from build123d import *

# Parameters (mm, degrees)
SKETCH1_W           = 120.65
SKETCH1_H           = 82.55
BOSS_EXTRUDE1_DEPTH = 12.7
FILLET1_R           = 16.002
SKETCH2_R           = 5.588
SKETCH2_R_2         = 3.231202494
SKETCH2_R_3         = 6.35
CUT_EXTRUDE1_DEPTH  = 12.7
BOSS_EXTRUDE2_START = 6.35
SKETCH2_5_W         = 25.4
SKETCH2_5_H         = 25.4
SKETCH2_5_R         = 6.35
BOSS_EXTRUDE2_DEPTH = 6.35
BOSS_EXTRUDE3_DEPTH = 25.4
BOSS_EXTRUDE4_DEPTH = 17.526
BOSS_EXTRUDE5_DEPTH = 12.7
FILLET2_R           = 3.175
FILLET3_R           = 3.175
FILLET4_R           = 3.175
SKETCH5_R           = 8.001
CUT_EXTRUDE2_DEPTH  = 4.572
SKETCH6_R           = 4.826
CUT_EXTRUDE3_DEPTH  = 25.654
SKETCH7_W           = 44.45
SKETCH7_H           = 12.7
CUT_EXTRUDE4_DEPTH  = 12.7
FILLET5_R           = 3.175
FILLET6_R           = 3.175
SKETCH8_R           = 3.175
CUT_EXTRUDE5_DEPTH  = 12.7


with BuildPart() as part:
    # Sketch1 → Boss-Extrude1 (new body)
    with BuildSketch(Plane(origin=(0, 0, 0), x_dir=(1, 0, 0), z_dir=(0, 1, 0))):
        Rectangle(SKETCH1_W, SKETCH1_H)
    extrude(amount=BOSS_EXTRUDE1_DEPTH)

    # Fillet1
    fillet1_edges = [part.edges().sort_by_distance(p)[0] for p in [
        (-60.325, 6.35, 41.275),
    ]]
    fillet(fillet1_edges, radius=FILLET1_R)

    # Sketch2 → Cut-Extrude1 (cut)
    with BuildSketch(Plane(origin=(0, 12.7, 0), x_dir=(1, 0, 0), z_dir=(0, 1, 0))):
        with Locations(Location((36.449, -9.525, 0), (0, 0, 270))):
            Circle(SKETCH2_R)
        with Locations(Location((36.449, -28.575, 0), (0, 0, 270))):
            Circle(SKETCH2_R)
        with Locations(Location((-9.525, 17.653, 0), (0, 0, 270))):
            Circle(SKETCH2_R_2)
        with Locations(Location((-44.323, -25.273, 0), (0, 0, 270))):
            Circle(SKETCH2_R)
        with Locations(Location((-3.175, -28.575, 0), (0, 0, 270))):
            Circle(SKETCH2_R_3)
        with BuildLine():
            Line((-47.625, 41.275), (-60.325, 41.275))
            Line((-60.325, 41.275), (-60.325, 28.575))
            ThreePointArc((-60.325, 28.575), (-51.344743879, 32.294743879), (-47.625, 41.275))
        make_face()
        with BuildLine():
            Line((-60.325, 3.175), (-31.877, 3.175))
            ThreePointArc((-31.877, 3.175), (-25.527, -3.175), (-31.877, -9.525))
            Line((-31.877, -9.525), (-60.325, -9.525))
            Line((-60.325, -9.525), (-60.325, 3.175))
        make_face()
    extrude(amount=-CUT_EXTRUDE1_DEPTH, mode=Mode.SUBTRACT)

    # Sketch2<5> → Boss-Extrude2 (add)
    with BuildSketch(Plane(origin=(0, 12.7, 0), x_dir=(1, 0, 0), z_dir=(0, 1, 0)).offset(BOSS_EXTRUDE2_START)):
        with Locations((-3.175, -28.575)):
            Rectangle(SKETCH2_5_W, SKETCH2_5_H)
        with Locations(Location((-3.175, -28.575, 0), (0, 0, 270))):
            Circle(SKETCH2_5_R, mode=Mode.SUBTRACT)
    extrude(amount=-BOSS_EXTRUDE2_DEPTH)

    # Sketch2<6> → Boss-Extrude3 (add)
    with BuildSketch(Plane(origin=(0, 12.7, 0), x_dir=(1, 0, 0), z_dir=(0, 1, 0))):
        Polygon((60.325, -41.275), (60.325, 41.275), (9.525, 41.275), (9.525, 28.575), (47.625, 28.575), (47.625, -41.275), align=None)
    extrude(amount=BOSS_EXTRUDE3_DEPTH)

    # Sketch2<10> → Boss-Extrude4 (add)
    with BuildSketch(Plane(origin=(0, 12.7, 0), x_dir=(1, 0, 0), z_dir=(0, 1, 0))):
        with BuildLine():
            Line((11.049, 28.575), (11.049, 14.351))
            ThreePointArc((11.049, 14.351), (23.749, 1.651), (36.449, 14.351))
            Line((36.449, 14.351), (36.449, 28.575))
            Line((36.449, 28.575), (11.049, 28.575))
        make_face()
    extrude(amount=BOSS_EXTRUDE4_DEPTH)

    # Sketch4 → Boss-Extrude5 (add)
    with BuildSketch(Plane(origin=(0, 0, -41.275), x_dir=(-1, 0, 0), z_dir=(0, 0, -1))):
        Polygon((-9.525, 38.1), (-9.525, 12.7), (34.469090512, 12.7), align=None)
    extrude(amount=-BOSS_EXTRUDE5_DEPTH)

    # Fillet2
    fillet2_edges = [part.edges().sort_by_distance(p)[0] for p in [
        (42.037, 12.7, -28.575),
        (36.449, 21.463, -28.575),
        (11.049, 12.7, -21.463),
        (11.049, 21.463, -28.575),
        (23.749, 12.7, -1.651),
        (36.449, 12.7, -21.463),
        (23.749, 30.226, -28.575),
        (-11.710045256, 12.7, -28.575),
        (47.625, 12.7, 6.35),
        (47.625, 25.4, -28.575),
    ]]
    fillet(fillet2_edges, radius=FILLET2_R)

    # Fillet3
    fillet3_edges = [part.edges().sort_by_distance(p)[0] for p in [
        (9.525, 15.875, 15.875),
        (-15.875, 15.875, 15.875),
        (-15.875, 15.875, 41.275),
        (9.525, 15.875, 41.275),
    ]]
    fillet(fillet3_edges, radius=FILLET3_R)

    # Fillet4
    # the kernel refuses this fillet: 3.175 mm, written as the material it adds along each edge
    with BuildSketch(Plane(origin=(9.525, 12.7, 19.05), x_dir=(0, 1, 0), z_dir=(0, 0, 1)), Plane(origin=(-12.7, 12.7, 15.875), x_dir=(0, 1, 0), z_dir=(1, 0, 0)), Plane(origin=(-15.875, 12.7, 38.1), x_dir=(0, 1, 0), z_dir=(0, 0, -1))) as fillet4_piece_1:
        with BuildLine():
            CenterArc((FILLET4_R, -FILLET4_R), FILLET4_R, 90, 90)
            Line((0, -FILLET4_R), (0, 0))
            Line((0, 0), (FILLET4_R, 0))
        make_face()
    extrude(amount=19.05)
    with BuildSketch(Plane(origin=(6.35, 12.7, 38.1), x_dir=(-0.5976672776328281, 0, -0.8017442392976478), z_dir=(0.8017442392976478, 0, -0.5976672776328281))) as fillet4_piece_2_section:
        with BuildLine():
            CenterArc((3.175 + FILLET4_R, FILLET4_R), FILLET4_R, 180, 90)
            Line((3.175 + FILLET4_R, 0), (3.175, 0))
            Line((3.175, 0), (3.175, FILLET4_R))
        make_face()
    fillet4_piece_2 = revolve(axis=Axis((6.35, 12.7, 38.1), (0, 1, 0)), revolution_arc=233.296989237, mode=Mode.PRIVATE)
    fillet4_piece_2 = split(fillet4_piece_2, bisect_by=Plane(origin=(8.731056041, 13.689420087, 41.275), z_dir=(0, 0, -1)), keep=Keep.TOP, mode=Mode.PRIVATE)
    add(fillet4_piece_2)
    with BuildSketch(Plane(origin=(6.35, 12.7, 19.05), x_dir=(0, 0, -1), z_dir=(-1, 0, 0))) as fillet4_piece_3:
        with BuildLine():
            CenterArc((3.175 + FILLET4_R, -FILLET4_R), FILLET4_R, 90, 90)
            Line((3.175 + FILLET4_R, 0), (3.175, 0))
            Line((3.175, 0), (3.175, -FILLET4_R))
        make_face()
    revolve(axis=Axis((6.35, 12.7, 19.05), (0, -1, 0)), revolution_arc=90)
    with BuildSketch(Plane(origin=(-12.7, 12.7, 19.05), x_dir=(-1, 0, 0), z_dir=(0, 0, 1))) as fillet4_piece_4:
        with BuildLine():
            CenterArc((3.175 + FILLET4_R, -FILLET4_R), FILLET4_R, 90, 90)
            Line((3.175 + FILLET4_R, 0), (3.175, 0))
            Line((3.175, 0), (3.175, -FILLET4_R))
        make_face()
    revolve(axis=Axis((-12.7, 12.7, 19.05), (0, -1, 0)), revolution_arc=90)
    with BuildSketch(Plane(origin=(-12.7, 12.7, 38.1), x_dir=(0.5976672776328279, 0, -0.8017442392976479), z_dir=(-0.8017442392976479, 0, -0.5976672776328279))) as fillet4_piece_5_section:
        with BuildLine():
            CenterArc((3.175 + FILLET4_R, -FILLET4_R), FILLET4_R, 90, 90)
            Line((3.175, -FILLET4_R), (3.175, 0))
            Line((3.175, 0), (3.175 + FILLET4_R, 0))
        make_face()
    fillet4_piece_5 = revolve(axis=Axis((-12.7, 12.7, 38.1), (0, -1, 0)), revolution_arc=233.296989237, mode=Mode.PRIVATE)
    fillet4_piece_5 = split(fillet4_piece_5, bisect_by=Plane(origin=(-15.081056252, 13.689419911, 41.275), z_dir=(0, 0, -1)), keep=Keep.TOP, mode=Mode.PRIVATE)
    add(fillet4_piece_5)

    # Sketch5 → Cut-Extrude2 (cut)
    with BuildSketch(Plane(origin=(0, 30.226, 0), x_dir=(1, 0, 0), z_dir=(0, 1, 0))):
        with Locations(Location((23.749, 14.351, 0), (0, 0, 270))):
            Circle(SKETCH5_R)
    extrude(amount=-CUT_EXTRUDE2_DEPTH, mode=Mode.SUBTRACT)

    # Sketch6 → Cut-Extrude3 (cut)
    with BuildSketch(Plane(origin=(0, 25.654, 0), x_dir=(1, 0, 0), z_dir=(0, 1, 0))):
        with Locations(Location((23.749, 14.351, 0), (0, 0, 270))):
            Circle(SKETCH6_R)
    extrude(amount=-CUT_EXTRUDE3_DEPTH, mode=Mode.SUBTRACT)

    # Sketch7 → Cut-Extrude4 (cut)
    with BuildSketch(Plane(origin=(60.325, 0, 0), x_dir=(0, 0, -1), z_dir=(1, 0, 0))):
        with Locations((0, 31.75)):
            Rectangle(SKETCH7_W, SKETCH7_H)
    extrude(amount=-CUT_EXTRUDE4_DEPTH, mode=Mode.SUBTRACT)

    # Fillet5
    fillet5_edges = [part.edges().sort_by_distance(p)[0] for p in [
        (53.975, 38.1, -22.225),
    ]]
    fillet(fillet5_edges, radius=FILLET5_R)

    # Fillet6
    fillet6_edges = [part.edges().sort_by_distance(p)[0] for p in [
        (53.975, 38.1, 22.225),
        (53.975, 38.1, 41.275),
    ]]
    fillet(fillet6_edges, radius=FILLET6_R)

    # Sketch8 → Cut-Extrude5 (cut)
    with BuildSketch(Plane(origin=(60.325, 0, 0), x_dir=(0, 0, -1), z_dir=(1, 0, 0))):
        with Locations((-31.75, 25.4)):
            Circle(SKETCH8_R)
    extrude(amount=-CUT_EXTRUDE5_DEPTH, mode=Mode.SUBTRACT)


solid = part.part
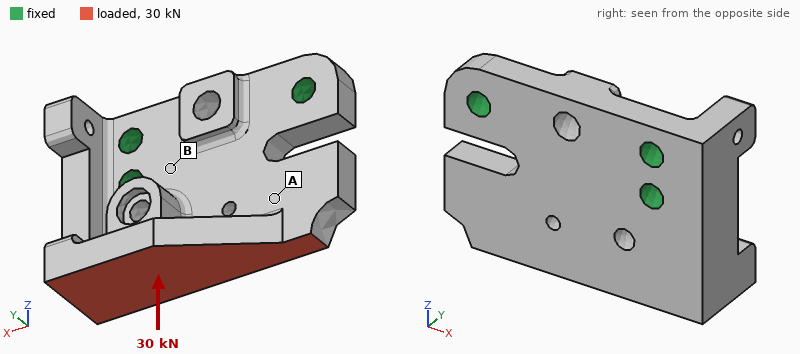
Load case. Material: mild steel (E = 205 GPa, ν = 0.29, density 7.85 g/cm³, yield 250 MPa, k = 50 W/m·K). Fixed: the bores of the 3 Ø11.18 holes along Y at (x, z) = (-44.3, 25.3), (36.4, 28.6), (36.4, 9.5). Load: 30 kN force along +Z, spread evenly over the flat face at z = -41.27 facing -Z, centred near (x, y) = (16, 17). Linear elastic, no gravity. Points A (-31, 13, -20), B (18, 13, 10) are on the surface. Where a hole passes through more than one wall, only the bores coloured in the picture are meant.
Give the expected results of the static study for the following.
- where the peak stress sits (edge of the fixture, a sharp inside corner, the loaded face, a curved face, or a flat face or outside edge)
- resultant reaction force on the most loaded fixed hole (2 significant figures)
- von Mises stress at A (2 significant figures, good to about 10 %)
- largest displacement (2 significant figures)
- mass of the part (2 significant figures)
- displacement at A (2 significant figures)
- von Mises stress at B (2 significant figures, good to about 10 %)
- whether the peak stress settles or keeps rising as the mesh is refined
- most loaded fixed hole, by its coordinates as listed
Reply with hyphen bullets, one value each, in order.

- edge of the fixture
- 16 kN
- 35 MPa
- 0.10 mm
- 1.3 kg
- 0.049 mm
- 74 MPa
- keeps rising
- (36.4, 9.5)
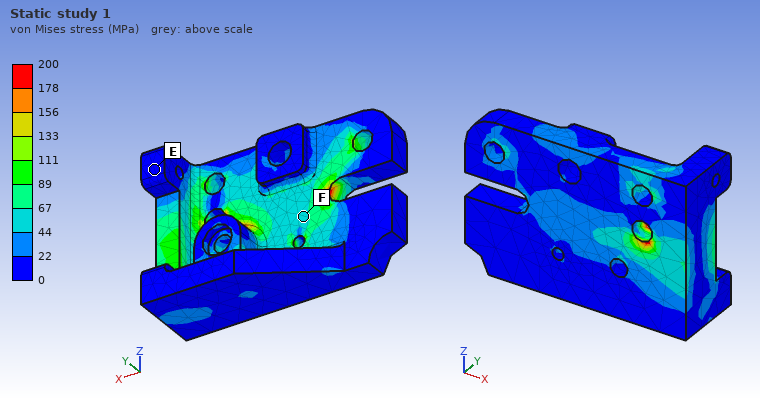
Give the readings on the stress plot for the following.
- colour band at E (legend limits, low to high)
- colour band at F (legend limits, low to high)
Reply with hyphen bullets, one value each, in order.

- 0 to 22 MPa
- 44 to 67 MPa
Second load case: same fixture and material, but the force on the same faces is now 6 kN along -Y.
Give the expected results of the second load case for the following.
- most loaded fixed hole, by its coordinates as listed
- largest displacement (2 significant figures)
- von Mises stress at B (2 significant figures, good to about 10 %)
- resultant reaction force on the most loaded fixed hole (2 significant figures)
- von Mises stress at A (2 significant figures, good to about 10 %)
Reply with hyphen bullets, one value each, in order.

- (36.4, 9.5)
- 0.11 mm
- 55 MPa
- 11 kN
- 13 MPa
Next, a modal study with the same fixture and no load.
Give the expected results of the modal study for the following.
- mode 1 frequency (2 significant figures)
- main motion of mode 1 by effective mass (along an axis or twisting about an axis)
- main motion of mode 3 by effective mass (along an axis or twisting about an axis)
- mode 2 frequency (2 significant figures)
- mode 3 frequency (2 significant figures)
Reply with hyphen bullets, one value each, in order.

- 2000 Hz
- along Y
- along X
- 3400 Hz
- 5200 Hz
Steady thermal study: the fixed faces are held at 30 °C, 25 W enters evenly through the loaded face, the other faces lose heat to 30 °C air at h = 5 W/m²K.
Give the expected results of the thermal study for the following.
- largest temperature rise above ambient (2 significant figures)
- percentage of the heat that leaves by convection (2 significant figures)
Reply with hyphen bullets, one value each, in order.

- 21 K
- 5.5 %
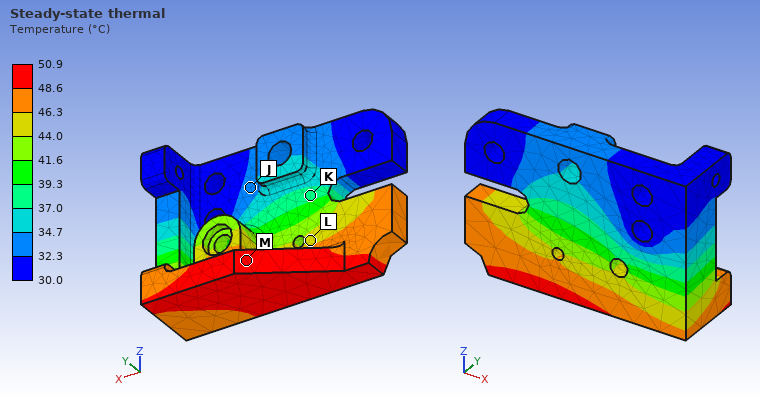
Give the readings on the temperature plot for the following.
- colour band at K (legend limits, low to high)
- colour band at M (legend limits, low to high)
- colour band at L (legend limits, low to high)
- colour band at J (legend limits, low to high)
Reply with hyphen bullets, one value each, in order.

- 37.0 to 39.3 °C
- 48.6 to 50.9 °C
- 44.0 to 46.3 °C
- 32.3 to 34.7 °C
